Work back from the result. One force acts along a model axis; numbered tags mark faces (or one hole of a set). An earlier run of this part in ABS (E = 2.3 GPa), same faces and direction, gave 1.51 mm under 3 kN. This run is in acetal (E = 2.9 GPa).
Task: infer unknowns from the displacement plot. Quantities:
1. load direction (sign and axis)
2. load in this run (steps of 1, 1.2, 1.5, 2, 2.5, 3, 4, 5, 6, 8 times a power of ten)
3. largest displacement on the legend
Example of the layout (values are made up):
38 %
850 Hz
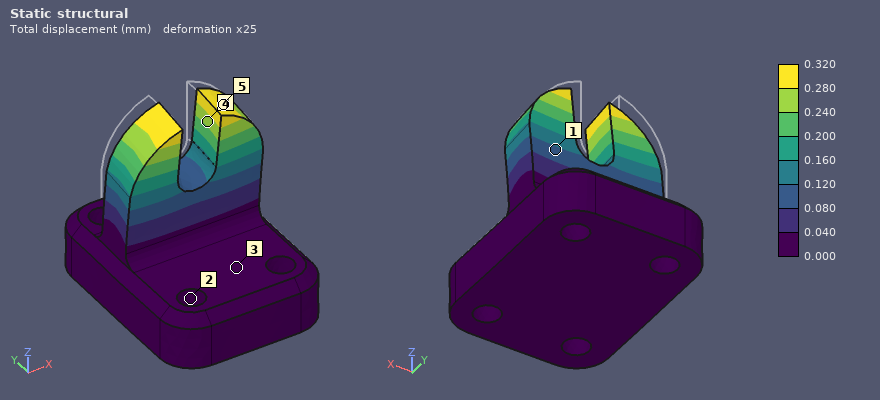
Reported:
-Y
800 N
0.320 mm
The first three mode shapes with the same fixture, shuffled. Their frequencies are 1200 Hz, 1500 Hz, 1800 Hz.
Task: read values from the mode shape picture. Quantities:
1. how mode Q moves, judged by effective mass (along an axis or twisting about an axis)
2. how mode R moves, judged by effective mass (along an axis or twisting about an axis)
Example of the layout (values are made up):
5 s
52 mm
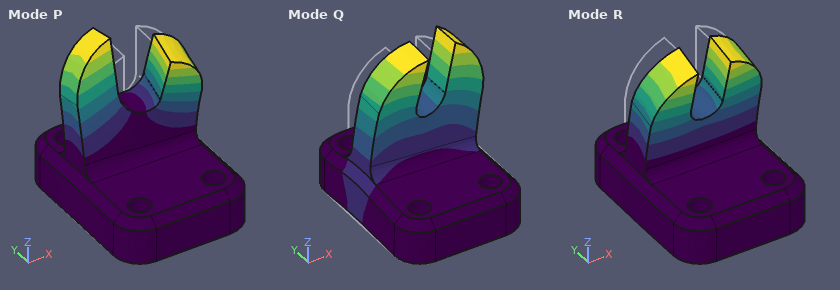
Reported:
along X
along Y
